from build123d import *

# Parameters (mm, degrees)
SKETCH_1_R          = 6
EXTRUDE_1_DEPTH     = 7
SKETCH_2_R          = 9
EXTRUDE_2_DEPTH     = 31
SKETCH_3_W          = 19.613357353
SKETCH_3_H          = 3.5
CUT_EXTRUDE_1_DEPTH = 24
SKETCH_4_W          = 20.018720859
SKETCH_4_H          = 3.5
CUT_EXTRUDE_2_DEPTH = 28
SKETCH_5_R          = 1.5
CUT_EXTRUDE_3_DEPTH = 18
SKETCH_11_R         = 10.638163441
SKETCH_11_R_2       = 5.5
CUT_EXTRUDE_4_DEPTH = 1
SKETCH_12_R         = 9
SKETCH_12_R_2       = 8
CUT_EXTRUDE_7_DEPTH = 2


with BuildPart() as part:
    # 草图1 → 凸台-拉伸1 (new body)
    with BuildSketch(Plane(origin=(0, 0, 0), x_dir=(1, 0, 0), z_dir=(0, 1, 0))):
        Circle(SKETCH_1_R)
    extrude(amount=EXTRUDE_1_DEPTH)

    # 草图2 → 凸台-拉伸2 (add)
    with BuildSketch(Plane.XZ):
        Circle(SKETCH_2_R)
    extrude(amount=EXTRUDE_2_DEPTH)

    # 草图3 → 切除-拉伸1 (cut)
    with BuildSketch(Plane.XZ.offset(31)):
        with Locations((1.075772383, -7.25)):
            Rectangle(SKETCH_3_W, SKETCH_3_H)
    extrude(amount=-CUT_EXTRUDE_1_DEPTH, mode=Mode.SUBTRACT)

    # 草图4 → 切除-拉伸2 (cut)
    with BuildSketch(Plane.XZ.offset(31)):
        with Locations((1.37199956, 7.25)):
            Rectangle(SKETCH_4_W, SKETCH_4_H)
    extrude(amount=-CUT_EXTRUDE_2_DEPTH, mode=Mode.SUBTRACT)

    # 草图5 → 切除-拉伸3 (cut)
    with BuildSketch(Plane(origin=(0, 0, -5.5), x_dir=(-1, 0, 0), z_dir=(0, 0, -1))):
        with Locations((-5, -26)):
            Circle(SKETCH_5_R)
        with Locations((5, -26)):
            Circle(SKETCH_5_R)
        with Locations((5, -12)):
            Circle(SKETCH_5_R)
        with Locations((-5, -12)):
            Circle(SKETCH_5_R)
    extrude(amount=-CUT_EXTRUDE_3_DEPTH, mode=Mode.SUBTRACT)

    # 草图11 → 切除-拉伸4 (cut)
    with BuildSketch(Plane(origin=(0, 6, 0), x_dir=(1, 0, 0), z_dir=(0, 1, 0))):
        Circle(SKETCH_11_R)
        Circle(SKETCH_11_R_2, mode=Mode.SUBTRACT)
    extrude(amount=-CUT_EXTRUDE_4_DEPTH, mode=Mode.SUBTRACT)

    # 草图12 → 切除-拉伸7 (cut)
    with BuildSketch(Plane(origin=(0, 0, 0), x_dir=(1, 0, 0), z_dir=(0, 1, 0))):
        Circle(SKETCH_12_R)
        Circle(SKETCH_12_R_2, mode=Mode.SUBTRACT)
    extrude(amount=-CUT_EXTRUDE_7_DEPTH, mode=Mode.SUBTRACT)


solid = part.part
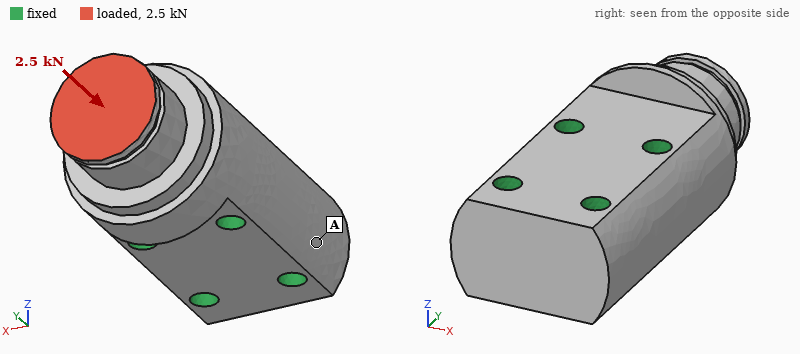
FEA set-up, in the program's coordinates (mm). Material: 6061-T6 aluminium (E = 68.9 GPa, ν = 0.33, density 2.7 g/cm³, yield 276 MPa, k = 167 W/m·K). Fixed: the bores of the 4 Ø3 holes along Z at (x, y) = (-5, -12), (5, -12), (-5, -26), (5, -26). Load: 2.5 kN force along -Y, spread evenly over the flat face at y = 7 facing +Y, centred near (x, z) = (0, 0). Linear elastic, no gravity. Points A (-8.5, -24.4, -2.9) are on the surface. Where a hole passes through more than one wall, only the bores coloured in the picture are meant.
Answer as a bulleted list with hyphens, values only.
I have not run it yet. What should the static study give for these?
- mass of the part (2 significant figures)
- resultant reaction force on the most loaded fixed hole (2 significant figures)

- 17 g
- 1.2 kN
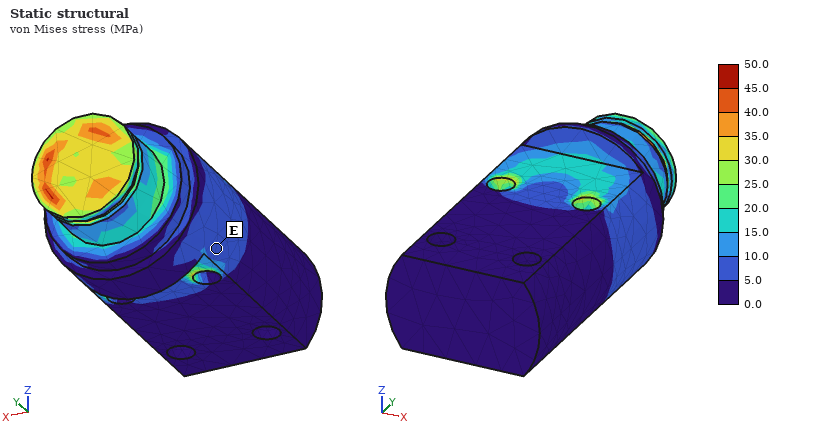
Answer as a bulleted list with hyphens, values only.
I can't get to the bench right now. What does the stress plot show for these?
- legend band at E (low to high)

- 5.0 to 10.0 MPa
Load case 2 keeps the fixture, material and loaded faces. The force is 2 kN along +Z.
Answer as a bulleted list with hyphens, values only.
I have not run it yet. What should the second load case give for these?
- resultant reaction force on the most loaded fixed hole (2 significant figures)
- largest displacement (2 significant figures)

- 1.1 kN
- 54 µm
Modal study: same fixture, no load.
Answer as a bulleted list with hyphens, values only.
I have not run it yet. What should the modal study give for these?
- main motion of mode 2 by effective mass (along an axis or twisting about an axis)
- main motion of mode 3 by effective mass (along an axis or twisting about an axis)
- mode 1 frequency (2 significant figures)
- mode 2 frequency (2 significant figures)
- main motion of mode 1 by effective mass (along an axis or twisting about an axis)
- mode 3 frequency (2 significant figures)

- along X
- twisting about Y
- 24 kHz
- 32 kHz
- along Z
- 49 kHz
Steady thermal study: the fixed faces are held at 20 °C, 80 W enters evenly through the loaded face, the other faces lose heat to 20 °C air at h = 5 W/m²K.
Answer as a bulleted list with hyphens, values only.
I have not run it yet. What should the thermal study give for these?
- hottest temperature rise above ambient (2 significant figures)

- 64 K
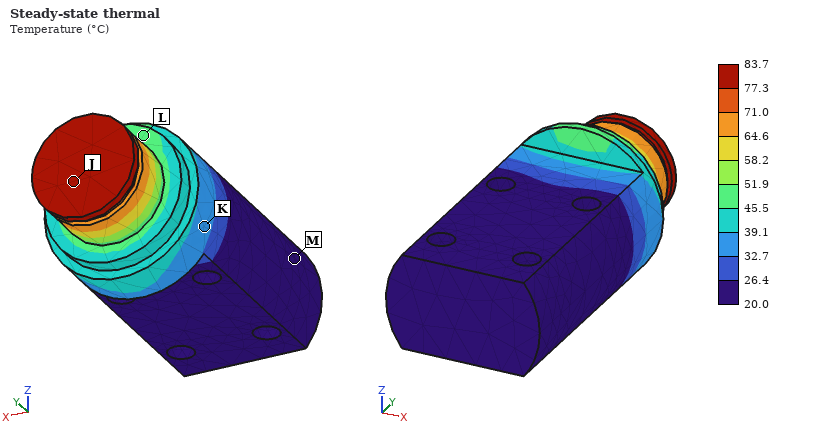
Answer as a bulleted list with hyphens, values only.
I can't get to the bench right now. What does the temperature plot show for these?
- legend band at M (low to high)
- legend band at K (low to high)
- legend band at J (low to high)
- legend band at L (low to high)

- 20.0 to 26.4 °C
- 32.7 to 39.1 °C
- 77.3 to 83.7 °C
- 45.5 to 51.9 °C
